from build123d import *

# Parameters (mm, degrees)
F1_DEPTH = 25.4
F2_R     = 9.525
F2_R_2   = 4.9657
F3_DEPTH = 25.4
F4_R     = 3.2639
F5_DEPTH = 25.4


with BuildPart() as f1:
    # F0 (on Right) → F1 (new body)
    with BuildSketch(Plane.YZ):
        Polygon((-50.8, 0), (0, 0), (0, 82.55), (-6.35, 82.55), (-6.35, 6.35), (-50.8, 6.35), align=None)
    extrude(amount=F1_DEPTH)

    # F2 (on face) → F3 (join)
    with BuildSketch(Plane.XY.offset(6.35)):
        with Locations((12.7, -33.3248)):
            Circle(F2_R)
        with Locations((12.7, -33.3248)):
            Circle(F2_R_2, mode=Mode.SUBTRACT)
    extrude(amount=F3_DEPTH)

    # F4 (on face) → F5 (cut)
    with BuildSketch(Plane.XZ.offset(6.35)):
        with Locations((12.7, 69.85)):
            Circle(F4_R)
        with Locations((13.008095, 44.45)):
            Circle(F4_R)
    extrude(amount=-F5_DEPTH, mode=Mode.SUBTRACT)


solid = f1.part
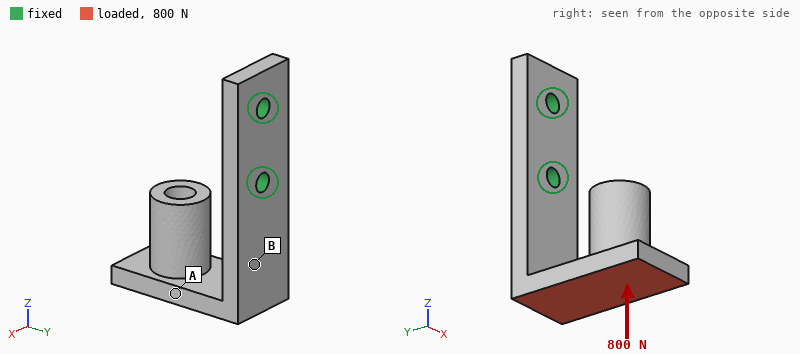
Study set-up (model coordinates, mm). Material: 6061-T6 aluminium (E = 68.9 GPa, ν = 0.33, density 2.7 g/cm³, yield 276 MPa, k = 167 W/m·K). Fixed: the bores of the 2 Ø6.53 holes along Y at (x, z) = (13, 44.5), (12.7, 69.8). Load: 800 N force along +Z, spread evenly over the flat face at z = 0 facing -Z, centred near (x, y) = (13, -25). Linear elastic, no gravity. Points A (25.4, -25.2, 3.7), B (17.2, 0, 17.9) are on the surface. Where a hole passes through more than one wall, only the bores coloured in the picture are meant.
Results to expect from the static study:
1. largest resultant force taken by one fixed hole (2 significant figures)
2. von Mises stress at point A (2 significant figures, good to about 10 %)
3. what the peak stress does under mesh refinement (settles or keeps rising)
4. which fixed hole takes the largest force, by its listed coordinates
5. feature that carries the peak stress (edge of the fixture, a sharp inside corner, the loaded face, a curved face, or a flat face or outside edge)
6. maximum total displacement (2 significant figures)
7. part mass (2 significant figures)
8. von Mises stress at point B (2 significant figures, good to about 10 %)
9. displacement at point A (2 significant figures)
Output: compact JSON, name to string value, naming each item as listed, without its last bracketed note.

{"largest resultant force taken by one fixed hole": "700 N", "von Mises stress at point A": "15 MPa", "what the peak stress does under mesh refinement": "keeps rising", "which fixed hole takes the largest force, by its listed coordinates": "(13, 44.5)", "feature that carries the peak stress": "edge of the fixture", "maximum total displacement": "1.2 mm", "part mass": "68 g", "von Mises stress at point B": "94 MPa", "displacement at point A": "0.60 mm"}
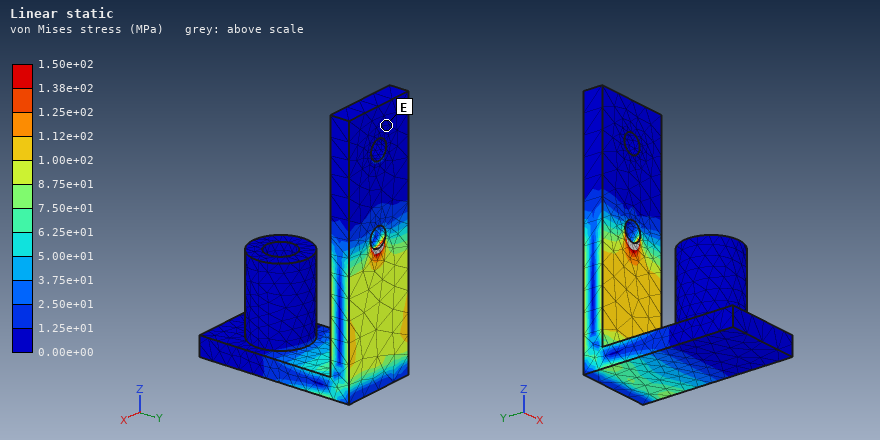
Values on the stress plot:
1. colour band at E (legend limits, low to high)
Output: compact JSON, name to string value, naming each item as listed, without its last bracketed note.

{"colour band at E": "0.00e+00 to 1.25e+01 MPa"}
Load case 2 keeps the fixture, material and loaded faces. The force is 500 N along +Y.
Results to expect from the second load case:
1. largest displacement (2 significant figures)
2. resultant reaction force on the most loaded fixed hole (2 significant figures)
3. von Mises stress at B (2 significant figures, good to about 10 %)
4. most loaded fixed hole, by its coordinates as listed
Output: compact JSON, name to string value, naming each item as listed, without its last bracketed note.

{"largest displacement": "0.72 mm", "resultant reaction force on the most loaded fixed hole": "660 N", "von Mises stress at B": "50 MPa", "most loaded fixed hole, by its coordinates as listed": "(13, 44.5)"}
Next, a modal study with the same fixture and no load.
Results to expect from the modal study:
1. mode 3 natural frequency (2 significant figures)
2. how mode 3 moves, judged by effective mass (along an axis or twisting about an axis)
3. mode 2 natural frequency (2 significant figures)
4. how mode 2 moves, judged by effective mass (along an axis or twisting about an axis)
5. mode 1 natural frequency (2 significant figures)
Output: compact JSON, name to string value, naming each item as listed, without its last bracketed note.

{"mode 3 natural frequency": "1700 Hz", "how mode 3 moves, judged by effective mass": "along Y", "mode 2 natural frequency": "980 Hz", "how mode 2 moves, judged by effective mass": "along X", "mode 1 natural frequency": "720 Hz"}
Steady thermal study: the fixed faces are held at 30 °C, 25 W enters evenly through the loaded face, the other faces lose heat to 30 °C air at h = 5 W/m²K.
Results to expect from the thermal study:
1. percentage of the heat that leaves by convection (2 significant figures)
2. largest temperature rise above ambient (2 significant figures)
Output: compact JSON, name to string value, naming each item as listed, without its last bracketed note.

{"percentage of the heat that leaves by convection": "5.1 %", "largest temperature rise above ambient": "53 K"}
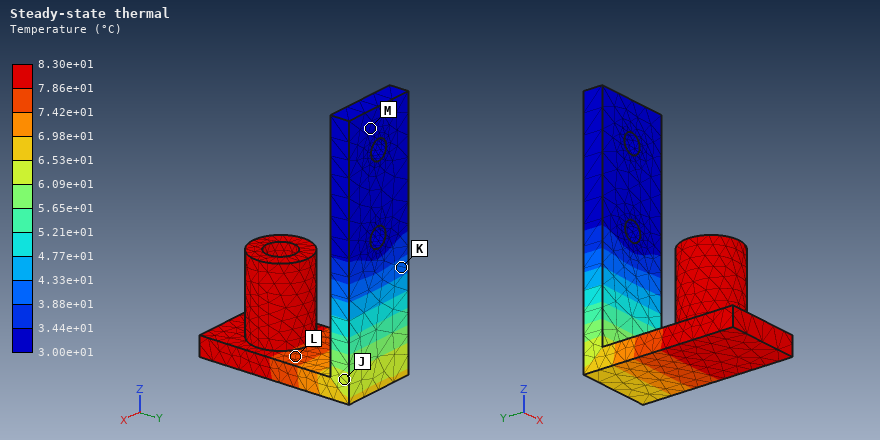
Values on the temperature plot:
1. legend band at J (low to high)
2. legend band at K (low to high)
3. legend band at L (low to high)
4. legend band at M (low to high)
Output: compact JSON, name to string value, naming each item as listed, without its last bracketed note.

{"legend band at J": "6.09e+01 to 6.53e+01 °C", "legend band at K": "3.88e+01 to 4.33e+01 °C", "legend band at L": "7.42e+01 to 7.86e+01 °C", "legend band at M": "3.00e+01 to 3.44e+01 °C"}
